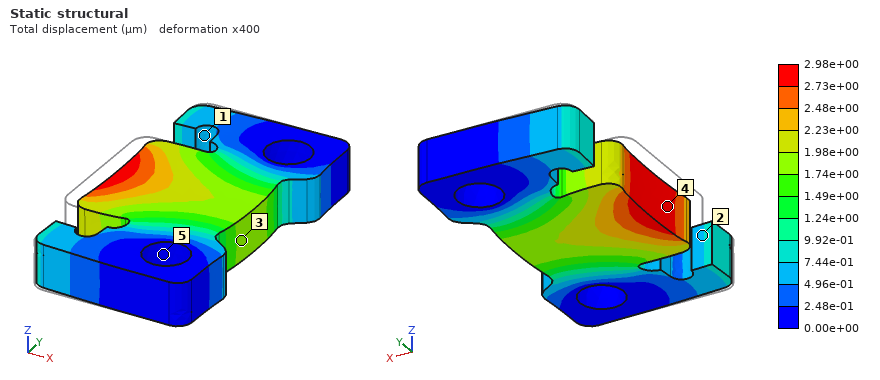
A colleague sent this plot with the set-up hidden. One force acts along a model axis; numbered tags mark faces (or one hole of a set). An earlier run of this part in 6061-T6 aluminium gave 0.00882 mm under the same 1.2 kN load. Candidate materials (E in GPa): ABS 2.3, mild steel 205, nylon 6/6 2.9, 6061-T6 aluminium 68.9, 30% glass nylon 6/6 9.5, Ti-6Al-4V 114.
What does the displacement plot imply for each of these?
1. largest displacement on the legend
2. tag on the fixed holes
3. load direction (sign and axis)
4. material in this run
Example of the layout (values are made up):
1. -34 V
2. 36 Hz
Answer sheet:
1. 2.98e+00 µm
2. 5
3. +X
4. mild steel
